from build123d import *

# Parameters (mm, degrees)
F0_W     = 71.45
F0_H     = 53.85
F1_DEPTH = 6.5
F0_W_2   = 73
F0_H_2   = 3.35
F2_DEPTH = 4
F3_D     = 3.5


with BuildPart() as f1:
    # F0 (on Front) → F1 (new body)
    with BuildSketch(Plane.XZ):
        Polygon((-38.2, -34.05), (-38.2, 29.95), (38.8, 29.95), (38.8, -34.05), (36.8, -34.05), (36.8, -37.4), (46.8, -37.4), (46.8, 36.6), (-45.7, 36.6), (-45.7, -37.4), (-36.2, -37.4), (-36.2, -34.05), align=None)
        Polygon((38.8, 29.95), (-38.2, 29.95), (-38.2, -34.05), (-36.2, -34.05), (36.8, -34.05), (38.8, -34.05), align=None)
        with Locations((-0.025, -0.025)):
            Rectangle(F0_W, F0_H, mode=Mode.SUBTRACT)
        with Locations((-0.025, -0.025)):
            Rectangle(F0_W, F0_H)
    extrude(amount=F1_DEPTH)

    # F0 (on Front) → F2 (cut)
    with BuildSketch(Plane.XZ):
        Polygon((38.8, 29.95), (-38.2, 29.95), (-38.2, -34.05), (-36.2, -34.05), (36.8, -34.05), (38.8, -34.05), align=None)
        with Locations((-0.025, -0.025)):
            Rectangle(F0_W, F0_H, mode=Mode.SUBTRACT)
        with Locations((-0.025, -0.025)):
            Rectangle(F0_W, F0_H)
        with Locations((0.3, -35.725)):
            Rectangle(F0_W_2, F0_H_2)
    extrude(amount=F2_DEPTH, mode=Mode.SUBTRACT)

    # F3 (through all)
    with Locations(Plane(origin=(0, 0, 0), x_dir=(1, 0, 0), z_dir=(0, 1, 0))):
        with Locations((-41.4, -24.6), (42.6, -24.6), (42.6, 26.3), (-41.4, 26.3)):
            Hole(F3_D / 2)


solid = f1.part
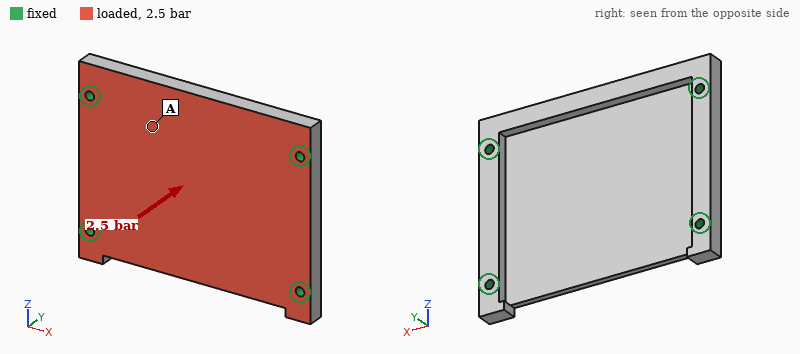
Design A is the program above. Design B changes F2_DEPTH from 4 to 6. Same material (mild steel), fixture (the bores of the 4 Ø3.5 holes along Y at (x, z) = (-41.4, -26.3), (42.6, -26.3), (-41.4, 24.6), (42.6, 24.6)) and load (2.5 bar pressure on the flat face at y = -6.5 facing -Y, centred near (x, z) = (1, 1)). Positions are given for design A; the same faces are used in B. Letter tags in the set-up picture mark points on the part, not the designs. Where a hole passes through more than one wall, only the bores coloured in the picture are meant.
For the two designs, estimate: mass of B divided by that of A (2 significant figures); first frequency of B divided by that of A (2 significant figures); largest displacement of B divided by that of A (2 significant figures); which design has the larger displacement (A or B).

0.57
0.24
97
B
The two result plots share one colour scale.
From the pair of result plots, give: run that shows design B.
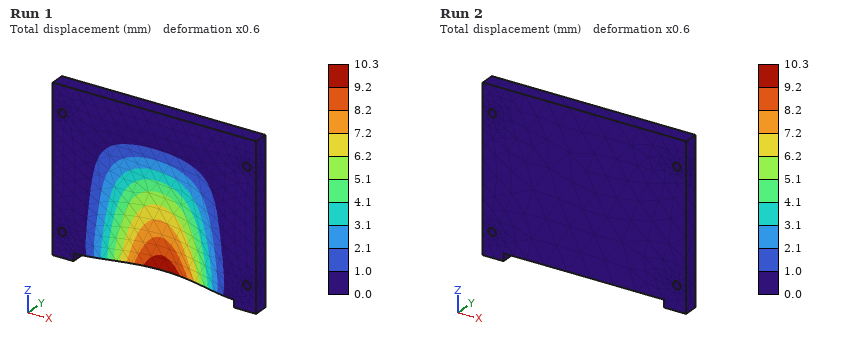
Run 1
